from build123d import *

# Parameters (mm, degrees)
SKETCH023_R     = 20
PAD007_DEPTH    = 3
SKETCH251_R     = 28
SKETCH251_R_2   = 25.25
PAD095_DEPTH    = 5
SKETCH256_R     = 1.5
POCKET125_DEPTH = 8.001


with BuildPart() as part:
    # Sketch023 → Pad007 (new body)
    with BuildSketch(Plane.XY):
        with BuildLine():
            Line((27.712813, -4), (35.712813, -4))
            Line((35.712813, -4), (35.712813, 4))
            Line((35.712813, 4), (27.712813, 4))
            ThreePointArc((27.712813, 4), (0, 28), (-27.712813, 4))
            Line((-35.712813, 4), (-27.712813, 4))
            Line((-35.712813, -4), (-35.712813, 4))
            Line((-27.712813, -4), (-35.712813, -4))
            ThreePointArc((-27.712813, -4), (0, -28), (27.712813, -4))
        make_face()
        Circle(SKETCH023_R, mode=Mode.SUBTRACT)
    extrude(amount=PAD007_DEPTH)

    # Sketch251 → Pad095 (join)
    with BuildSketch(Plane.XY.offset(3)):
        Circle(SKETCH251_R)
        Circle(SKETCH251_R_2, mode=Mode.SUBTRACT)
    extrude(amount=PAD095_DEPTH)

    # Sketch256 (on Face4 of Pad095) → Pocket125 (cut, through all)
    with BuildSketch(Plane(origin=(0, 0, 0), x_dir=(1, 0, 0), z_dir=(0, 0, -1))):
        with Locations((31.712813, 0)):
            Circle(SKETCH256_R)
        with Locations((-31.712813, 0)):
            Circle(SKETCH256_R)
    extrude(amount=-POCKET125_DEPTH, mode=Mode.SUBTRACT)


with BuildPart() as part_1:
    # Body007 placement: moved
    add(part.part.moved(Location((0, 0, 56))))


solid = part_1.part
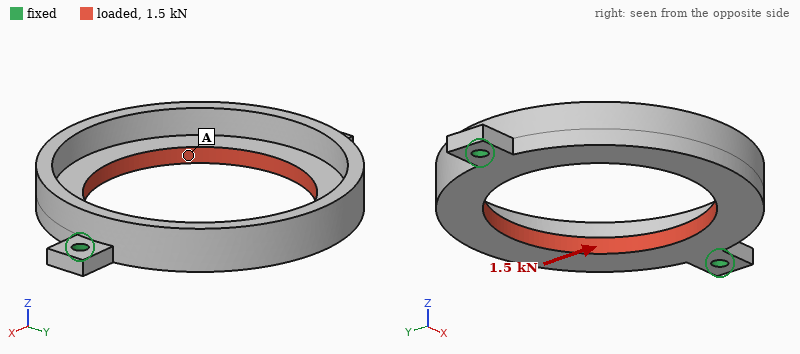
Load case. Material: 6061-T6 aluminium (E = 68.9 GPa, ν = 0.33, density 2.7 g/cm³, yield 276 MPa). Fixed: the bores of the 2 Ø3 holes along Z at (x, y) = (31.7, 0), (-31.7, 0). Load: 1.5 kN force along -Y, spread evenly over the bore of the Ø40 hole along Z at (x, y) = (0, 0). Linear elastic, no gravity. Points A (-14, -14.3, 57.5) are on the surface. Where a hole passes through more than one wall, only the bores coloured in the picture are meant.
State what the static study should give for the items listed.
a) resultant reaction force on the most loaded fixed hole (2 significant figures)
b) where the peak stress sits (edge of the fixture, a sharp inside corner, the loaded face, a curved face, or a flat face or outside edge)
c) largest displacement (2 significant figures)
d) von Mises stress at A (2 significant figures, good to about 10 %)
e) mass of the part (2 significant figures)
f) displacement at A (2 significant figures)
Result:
750 N
edge of the fixture
25 µm
16 MPa
17 g
14 µm
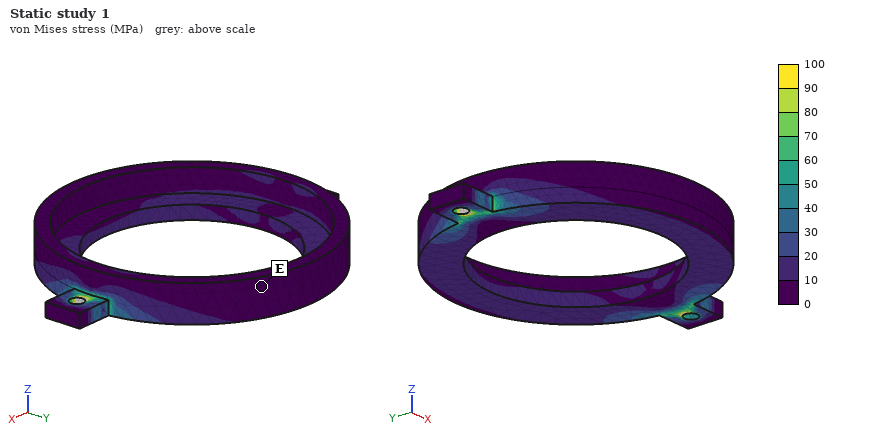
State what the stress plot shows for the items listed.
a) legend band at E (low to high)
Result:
0 to 10 MPa
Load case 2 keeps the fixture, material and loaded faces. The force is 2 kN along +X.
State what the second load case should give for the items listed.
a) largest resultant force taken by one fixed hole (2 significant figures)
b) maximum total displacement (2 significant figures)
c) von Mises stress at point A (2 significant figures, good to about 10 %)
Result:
1.0 kN
34 µm
54 MPa
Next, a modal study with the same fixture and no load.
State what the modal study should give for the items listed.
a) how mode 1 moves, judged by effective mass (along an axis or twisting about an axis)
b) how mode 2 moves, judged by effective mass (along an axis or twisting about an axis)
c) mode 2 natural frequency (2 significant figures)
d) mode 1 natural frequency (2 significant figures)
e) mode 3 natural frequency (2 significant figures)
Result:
twisting about X
along Z
3100 Hz
1800 Hz
6100 Hz
